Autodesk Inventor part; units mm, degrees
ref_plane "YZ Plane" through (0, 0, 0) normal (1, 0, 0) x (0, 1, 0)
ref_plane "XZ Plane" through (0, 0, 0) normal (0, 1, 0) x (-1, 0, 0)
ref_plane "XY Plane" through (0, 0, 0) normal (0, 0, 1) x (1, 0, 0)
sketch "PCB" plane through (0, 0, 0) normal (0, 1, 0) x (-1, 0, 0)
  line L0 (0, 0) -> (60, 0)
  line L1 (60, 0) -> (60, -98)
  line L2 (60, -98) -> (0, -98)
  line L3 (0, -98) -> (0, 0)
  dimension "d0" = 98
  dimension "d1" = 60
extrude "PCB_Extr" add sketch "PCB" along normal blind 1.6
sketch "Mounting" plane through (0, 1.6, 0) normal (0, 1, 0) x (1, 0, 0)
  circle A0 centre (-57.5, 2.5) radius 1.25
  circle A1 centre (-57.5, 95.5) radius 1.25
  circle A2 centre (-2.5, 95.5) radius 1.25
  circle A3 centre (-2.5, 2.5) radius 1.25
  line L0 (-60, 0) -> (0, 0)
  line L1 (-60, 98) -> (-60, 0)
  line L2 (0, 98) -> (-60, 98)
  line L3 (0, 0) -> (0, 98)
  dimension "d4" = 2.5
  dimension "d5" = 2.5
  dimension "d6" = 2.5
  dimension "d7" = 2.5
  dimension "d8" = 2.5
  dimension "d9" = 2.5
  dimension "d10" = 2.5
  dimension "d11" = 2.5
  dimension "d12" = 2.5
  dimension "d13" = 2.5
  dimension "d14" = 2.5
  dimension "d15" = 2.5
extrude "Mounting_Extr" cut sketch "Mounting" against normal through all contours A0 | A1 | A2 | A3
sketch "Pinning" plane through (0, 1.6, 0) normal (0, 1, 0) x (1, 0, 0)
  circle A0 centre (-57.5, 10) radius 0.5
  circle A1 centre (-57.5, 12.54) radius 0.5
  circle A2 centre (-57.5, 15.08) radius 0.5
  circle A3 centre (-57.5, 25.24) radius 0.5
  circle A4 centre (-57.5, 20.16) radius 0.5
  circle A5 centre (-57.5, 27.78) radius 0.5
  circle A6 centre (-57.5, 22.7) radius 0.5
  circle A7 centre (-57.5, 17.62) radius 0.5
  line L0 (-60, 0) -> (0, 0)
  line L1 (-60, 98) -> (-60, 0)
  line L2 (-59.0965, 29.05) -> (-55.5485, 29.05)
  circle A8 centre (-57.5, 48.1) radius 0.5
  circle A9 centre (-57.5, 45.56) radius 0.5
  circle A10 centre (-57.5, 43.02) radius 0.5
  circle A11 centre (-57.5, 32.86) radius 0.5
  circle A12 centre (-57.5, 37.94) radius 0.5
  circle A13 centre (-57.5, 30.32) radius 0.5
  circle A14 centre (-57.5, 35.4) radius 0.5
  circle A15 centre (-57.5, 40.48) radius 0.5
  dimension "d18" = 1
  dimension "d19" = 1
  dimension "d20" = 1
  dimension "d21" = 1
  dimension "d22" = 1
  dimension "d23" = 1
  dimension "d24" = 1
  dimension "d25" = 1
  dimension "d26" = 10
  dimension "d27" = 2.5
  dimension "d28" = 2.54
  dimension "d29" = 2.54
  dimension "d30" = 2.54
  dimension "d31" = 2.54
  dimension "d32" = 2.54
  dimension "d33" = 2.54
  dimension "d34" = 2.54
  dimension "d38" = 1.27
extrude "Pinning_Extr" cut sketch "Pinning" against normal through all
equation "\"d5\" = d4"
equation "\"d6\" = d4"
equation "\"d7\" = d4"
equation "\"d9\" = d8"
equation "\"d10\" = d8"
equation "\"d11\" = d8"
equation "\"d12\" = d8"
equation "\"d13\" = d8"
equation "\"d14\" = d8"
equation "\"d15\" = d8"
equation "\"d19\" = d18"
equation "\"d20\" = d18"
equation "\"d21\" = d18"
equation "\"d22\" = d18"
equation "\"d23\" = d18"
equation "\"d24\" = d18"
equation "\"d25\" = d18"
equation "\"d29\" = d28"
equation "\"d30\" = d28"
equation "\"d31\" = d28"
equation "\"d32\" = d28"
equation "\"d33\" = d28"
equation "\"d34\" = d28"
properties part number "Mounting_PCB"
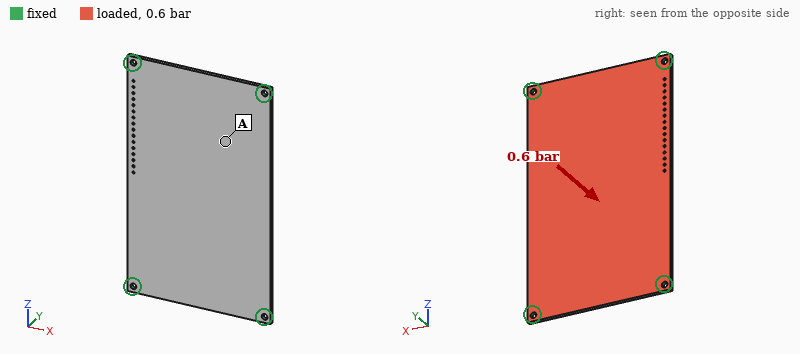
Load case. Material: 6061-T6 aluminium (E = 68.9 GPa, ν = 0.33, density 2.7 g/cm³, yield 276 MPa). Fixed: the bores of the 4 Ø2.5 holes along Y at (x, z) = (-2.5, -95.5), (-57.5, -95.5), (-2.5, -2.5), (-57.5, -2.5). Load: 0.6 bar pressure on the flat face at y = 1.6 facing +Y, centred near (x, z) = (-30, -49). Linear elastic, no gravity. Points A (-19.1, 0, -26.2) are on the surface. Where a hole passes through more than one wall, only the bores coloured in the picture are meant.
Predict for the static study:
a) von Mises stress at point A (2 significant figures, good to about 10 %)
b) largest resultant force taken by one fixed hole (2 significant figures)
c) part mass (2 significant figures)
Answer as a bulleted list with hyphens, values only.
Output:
- 32 MPa
- 88 N
- 25 g
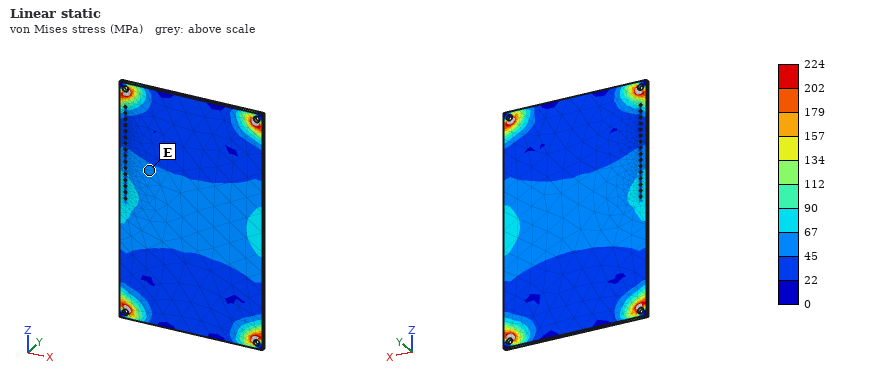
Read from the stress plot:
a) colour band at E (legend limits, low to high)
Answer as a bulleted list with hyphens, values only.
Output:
- 45 to 67 MPa
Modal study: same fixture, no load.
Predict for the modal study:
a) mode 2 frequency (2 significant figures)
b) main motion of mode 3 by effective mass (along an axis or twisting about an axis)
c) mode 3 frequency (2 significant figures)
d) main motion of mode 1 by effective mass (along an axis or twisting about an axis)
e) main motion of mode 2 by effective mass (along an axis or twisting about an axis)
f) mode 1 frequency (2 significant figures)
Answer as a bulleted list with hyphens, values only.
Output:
- 1300 Hz
- twisting about X
- 2000 Hz
- along Y
- twisting about Z
- 750 Hz
